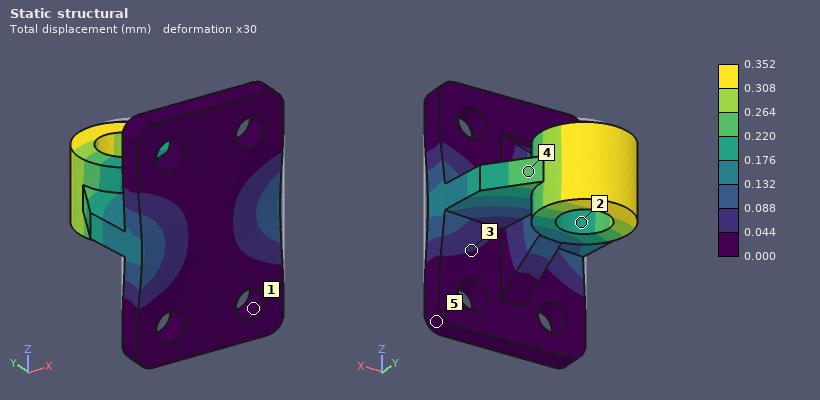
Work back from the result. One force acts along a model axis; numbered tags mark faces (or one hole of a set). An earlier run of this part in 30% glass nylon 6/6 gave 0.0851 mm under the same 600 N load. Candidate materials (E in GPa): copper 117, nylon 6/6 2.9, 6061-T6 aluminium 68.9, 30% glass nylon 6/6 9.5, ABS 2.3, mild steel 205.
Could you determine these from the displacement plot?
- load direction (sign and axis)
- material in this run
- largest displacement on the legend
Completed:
-X
ABS
0.352 mm
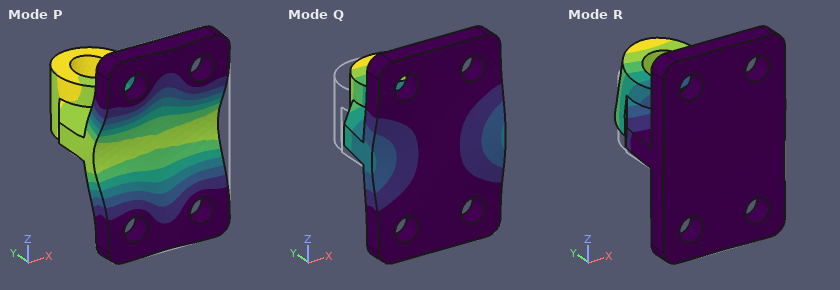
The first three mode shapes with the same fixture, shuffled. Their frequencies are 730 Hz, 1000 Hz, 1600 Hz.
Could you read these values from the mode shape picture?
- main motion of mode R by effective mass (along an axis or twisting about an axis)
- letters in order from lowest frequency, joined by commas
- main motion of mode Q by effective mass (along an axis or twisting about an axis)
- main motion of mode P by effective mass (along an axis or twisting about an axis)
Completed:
along Z
Q, R, P
along X
along Y
